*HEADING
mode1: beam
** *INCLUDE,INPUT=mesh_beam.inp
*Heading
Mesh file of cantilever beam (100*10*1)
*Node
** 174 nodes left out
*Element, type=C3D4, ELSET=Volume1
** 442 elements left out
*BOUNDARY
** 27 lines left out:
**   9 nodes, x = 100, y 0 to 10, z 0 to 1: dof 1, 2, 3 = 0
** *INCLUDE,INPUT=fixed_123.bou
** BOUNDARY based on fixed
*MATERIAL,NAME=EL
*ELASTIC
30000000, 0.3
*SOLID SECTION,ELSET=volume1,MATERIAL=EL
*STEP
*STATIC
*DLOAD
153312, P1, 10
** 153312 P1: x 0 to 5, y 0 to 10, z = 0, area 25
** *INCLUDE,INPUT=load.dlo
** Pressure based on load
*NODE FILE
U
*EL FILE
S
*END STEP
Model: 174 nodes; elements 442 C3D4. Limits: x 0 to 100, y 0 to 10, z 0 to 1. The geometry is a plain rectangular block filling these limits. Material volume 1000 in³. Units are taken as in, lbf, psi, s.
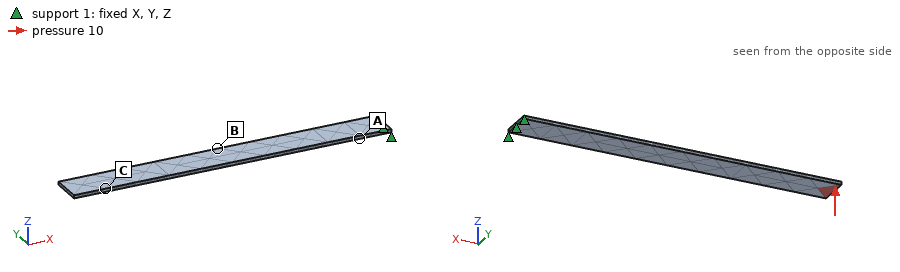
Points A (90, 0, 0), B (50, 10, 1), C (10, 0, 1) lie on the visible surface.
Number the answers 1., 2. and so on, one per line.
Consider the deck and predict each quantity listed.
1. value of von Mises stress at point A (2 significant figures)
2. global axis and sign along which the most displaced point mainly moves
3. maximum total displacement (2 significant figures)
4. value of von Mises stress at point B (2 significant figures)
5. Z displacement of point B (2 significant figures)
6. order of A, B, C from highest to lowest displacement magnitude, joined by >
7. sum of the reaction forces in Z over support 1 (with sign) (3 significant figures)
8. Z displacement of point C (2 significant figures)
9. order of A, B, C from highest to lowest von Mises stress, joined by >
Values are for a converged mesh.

1. 13000 psi
2. +Z
3. 3.2 in
4. 7300 psi
5. 0.99 in
6. C > B > A
7. -250 lbf
8. 2.7 in
9. A > B > C
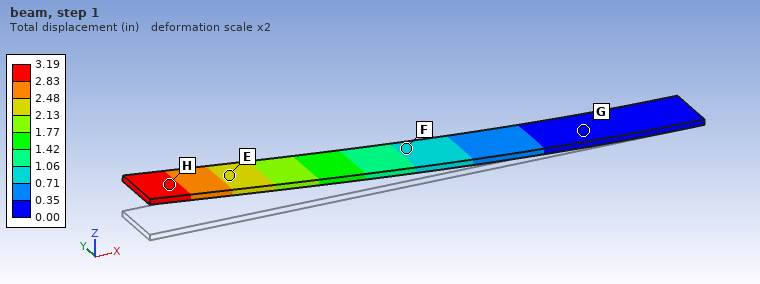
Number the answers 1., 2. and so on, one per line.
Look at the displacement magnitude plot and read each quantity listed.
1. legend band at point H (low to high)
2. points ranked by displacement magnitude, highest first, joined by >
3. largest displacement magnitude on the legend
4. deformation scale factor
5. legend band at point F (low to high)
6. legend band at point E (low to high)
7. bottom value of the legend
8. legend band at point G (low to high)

1. 2.83 to 3.19 in
2. H > E > F > G
3. 3.19 in
4. 2
5. 0.71 to 1.06 in
6. 2.13 to 2.48 in
7. 0.00 in
8. 0.00 to 0.35 in
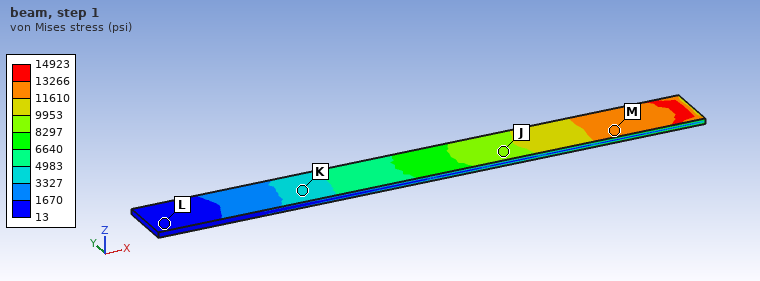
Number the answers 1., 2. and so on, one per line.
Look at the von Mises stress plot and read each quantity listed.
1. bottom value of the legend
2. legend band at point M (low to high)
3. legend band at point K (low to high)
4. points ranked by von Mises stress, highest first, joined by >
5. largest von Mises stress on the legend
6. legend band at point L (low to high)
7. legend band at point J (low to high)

1. 13 psi
2. 11610 to 13266 psi
3. 3327 to 4983 psi
4. M > J > K > L
5. 14923 psi
6. 13 to 1670 psi
7. 8297 to 9953 psi
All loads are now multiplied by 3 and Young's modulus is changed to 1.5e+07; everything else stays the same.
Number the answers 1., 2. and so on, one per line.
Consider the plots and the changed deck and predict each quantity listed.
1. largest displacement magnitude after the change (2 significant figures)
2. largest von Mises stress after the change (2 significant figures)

1. 19 in
2. 45000 psi
